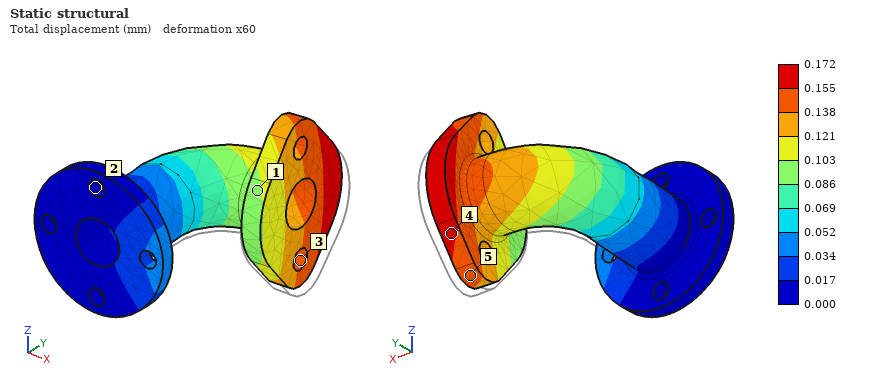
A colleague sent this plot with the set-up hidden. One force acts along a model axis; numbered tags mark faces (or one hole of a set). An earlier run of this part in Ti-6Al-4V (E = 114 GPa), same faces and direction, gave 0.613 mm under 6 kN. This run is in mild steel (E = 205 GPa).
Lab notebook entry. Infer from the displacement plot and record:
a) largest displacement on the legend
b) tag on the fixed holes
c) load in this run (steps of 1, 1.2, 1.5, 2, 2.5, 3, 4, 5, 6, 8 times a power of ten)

0.172 mm
2
3 kN
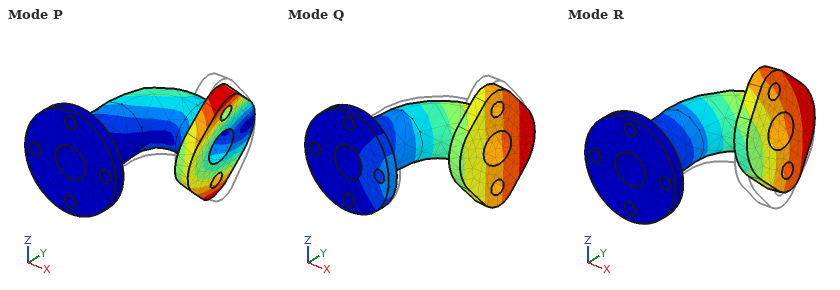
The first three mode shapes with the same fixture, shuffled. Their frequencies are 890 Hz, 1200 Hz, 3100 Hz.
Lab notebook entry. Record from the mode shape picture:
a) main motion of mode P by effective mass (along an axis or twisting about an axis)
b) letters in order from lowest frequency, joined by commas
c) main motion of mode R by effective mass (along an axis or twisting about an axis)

twisting about Y
Q, R, P
along Z
